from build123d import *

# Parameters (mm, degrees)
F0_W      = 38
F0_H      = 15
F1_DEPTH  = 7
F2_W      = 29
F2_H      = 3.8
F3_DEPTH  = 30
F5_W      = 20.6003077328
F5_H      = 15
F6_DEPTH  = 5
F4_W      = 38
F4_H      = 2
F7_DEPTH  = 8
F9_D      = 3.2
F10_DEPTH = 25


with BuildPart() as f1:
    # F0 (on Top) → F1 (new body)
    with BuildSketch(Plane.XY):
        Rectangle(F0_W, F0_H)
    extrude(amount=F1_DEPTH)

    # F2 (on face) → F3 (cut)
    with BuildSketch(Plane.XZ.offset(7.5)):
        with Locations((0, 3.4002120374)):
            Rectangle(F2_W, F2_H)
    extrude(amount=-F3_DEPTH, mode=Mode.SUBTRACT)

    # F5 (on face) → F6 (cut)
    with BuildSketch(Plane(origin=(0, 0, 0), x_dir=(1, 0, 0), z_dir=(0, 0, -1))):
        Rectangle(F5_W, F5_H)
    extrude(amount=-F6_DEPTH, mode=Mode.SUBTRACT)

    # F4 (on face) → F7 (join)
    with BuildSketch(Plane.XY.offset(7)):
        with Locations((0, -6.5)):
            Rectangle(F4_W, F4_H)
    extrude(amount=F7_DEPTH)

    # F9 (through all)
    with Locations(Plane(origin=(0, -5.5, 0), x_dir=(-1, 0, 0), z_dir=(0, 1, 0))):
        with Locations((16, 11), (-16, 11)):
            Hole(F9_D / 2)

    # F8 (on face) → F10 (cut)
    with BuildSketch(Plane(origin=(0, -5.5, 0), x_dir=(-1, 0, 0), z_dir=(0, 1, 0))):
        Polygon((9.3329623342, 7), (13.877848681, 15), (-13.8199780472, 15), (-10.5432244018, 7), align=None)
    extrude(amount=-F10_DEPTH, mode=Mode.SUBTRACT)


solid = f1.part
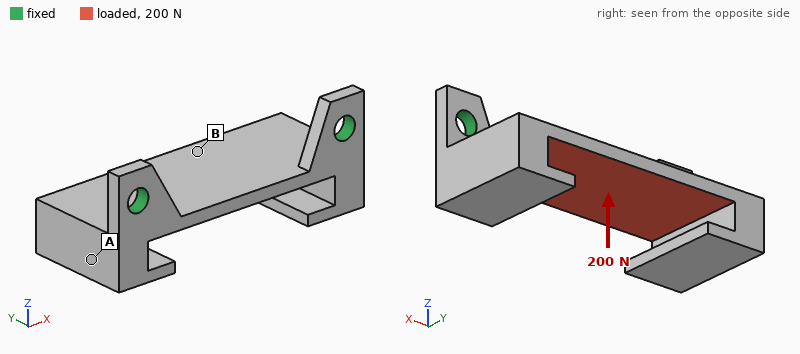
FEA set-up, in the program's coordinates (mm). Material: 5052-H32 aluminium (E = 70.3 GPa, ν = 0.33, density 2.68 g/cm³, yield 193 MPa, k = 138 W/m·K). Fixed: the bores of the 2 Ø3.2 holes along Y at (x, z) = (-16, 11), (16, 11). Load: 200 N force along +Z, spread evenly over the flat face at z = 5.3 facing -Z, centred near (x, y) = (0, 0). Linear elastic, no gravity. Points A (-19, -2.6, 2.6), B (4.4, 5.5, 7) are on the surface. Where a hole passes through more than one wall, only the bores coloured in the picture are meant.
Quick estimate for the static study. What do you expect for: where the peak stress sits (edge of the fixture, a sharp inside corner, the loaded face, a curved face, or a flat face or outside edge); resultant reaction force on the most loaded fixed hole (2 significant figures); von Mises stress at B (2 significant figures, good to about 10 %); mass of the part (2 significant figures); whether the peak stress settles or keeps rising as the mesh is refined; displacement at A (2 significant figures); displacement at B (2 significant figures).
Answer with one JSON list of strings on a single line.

["edge of the fixture", "120 N", "30 MPa", "5.5 g", "keeps rising", "0.044 mm", "0.12 mm"]
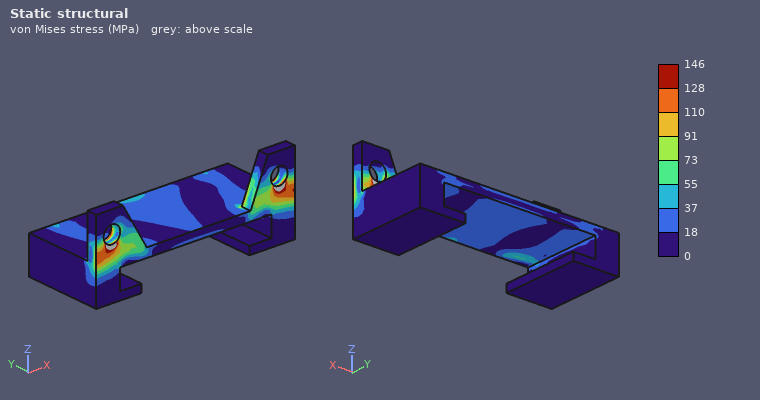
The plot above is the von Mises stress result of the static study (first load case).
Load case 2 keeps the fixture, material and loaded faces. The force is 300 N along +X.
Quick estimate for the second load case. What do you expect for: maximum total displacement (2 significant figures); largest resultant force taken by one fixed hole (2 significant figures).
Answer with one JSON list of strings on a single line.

["11 µm", "160 N"]
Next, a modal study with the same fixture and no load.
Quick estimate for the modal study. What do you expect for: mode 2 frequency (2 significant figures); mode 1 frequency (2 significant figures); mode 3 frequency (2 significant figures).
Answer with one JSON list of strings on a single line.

["4700 Hz", "3300 Hz", "10 kHz"]
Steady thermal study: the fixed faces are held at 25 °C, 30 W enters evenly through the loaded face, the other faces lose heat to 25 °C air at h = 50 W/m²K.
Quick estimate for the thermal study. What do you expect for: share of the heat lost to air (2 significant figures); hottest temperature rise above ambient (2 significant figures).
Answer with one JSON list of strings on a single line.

["10 %", "61 K"]
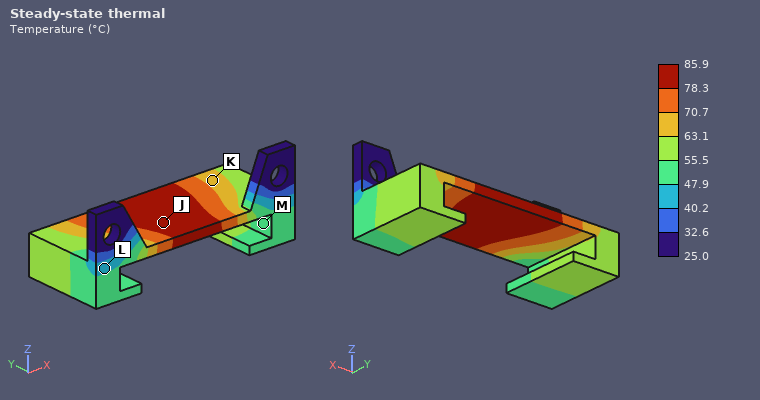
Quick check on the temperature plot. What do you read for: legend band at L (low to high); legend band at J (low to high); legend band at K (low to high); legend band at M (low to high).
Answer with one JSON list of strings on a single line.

["40.2 to 47.9 °C", "78.3 to 85.9 °C", "63.1 to 70.7 °C", "47.9 to 55.5 °C"]
